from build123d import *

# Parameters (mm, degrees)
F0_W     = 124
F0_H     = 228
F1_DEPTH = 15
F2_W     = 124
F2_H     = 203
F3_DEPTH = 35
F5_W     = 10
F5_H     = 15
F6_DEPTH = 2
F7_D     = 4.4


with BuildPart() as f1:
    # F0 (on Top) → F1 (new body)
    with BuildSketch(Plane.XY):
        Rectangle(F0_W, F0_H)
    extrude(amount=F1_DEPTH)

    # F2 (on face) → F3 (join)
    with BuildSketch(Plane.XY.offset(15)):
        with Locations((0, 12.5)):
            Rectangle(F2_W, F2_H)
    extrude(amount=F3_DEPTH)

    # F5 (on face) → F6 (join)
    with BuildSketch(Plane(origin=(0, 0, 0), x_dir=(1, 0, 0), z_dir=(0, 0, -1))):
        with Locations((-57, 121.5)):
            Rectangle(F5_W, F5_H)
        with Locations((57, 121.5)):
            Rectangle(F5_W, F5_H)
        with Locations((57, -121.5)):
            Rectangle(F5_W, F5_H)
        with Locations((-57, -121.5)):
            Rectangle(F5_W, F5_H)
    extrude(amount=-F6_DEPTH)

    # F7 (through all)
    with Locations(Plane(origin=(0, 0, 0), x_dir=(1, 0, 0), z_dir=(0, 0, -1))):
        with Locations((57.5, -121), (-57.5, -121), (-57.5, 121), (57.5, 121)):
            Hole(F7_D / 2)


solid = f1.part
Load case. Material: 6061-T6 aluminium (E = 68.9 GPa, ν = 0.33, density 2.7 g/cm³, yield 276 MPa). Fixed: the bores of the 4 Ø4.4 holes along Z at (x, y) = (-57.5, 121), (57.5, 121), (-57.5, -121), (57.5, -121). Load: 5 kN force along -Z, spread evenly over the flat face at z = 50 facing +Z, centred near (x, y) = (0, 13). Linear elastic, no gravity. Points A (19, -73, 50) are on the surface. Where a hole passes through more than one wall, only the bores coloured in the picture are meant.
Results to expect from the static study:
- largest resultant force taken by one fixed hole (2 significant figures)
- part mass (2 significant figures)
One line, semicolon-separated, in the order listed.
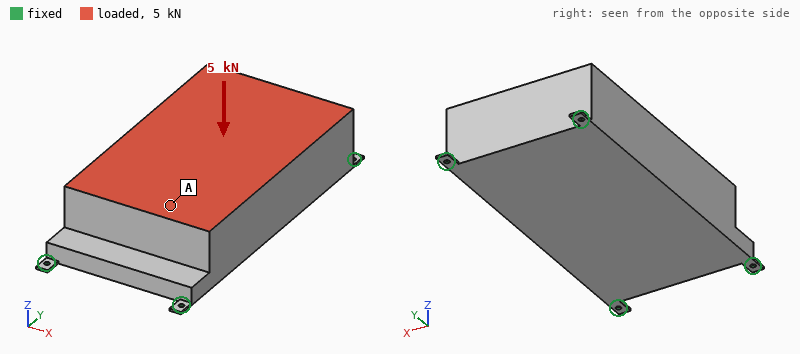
1.7 kN; 3.5 kg
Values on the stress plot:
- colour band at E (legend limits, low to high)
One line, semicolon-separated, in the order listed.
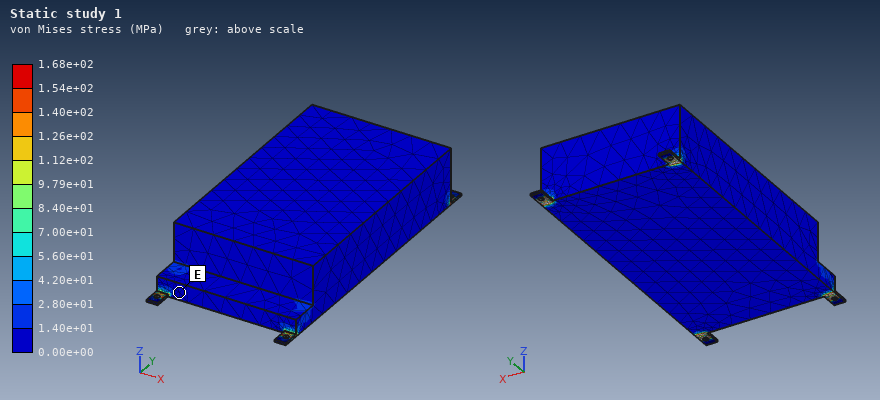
0.00e+00 to 1.40e+01 MPa
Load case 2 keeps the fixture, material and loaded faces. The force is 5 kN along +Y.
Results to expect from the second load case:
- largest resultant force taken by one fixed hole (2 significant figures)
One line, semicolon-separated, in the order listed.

1.4 kN
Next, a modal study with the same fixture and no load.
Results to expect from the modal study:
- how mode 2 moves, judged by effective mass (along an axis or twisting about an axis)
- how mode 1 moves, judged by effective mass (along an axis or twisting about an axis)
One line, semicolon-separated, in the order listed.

along X; along Z
